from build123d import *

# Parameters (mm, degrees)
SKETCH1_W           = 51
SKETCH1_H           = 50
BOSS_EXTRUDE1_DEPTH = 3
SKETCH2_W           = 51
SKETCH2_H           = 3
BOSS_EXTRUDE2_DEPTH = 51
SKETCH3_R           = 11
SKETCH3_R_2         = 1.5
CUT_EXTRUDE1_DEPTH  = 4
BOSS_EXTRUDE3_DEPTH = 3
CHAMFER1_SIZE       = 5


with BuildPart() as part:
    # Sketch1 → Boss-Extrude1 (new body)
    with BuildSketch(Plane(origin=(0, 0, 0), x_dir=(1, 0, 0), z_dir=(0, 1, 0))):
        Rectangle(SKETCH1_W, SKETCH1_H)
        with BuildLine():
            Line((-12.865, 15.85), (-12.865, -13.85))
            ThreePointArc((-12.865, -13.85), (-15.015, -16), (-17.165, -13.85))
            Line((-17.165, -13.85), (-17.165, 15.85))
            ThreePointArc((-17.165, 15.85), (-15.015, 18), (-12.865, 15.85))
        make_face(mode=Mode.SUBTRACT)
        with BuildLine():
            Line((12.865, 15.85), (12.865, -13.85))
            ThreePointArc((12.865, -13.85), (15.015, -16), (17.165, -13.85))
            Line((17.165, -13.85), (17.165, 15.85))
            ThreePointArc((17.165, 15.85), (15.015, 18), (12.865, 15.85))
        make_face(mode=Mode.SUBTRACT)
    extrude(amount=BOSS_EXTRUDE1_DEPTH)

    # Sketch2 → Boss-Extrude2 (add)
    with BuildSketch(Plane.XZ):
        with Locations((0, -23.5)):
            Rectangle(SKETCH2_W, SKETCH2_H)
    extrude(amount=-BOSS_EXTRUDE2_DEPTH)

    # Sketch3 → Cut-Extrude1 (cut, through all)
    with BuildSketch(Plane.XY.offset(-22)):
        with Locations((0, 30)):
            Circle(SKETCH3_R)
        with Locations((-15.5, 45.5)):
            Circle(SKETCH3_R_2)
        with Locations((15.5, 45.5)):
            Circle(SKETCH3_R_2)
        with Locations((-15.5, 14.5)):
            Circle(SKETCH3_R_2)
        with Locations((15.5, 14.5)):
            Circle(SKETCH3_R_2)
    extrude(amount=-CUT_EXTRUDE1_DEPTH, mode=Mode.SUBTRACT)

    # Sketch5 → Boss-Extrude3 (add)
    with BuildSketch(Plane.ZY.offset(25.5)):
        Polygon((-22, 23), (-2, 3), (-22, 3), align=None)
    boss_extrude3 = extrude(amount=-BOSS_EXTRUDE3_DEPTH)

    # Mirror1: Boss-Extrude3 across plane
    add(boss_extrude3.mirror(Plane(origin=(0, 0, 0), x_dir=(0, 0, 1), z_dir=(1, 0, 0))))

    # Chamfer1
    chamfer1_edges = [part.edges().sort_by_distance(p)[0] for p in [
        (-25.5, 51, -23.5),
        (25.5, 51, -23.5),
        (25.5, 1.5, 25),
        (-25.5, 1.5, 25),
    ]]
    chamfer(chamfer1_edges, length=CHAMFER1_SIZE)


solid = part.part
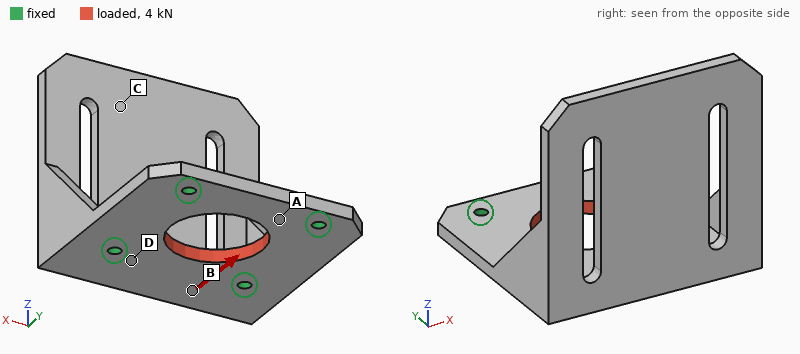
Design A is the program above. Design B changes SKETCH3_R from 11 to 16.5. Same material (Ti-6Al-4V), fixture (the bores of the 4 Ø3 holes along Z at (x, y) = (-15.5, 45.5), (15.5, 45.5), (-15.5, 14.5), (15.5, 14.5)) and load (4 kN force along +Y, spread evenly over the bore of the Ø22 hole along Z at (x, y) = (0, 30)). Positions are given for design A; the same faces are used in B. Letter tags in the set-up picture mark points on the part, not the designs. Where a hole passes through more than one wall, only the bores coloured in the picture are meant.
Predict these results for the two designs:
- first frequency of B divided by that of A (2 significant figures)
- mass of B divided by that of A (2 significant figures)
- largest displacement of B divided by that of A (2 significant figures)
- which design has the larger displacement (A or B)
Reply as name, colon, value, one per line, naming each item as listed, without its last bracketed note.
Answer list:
first frequency of B divided by that of A: 0.98
mass of B divided by that of A: 0.90
largest displacement of B divided by that of A: 1.8
which design has the larger displacement: B
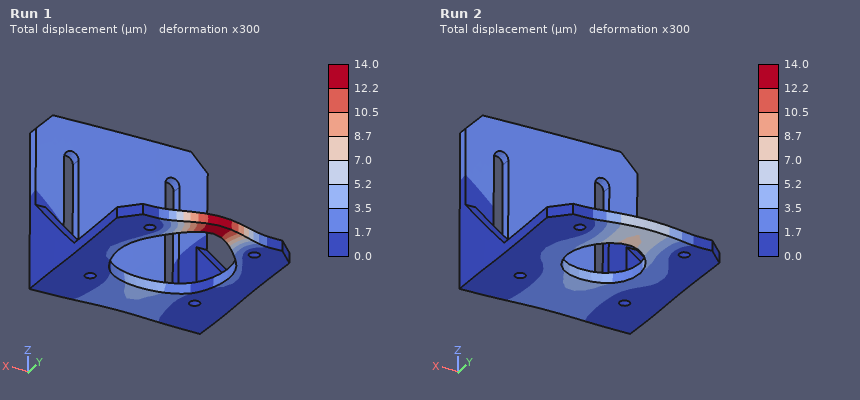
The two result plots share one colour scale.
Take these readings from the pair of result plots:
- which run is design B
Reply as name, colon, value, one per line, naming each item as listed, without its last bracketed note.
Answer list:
which run is design B: Run 1
